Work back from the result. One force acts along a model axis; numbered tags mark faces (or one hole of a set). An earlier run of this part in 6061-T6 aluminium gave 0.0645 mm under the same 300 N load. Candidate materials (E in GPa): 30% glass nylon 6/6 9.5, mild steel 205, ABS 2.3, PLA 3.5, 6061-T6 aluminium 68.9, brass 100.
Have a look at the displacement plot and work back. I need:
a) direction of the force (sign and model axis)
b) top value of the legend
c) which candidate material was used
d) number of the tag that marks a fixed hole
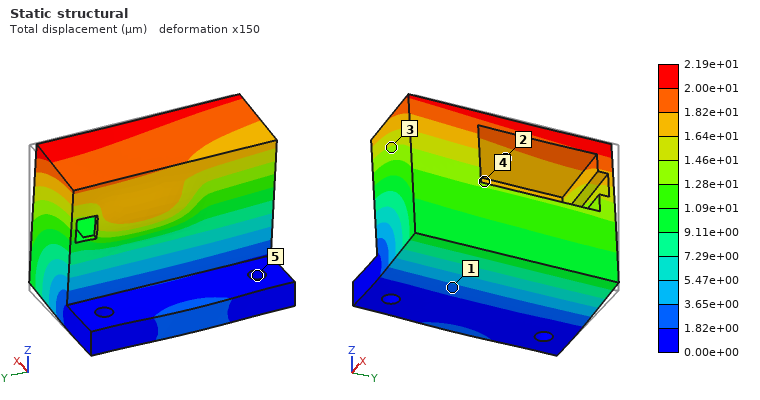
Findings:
-X
2.19e+01 µm
mild steel
5
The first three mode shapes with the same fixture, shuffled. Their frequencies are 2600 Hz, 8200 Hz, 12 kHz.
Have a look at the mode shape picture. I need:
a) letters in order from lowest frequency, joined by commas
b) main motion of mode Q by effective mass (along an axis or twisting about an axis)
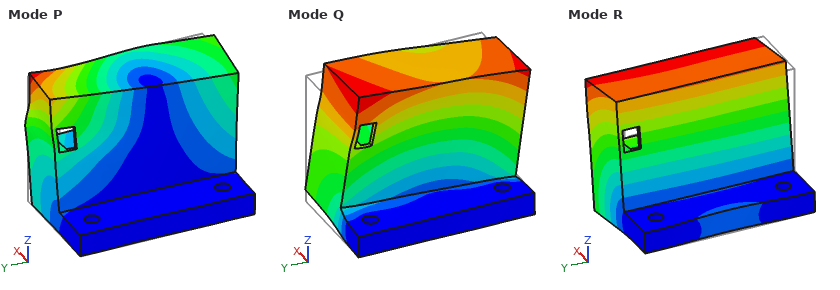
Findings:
R, Q, P
along Y
